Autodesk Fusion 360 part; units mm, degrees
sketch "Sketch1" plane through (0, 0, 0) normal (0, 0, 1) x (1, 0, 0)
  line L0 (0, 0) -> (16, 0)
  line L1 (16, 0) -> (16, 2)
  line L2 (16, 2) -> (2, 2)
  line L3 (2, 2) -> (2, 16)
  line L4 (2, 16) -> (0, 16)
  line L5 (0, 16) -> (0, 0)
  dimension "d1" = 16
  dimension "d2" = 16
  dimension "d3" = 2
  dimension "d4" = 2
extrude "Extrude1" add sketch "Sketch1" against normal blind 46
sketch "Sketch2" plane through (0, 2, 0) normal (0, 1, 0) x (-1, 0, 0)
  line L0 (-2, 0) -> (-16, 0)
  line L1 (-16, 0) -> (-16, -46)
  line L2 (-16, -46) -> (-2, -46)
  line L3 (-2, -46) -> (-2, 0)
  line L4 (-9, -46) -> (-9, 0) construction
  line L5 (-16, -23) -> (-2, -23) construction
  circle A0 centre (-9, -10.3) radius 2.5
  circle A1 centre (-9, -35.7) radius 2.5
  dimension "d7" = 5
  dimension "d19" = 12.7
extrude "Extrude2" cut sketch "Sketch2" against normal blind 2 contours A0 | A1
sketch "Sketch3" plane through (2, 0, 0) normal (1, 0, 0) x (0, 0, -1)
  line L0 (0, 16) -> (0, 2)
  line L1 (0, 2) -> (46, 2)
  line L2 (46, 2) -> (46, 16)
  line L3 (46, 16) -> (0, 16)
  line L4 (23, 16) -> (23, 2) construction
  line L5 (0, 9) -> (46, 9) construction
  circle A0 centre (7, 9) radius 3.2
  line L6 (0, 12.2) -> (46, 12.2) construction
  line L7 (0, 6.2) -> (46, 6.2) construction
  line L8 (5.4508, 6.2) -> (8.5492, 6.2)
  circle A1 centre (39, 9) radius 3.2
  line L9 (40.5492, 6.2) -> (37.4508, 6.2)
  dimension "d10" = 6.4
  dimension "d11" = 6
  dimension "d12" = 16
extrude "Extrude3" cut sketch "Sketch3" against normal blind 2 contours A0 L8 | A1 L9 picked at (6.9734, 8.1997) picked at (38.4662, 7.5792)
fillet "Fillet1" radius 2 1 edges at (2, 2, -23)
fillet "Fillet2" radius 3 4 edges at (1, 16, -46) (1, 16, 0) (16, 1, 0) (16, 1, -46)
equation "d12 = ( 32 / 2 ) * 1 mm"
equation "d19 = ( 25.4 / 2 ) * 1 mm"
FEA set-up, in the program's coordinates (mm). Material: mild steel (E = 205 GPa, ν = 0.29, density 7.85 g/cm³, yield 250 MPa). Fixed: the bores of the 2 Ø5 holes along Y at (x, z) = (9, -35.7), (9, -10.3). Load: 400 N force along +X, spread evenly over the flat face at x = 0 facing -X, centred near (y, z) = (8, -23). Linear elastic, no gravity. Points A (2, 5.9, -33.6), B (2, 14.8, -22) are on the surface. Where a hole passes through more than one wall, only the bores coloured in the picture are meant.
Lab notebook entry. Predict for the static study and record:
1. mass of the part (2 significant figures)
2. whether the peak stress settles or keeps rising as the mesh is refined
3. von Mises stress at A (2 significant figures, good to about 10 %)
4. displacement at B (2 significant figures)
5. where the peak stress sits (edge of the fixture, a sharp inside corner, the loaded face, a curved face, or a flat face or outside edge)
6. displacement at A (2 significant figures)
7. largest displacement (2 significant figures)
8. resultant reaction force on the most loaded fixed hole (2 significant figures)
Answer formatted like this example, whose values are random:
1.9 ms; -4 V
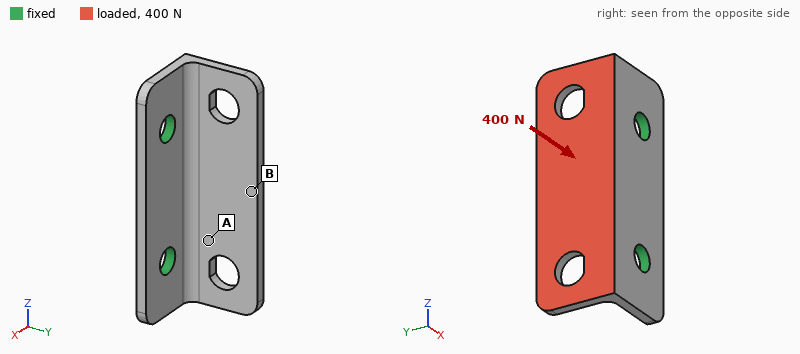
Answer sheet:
20 g; keeps rising; 44 MPa; 52 µm; edge of the fixture; 16 µm; 59 µm; 200 N
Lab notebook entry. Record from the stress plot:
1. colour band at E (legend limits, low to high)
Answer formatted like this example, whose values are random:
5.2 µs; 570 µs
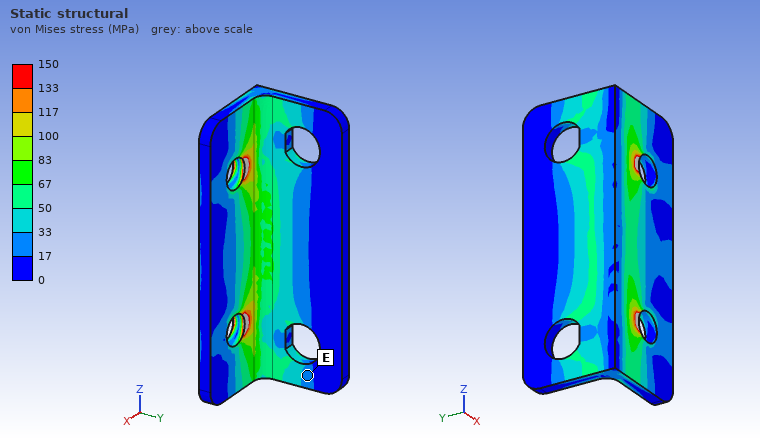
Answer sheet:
17 to 33 MPa
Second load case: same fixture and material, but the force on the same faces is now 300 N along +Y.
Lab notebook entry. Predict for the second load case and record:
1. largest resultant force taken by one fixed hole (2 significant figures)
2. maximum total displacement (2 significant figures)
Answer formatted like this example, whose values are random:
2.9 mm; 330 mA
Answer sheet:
150 N; 26 µm
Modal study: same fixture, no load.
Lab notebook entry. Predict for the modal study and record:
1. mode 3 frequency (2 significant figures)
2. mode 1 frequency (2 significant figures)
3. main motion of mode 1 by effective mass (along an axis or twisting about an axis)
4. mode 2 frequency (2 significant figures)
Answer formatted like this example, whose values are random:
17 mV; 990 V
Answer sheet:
13 kHz; 4700 Hz; along X; 6900 Hz
